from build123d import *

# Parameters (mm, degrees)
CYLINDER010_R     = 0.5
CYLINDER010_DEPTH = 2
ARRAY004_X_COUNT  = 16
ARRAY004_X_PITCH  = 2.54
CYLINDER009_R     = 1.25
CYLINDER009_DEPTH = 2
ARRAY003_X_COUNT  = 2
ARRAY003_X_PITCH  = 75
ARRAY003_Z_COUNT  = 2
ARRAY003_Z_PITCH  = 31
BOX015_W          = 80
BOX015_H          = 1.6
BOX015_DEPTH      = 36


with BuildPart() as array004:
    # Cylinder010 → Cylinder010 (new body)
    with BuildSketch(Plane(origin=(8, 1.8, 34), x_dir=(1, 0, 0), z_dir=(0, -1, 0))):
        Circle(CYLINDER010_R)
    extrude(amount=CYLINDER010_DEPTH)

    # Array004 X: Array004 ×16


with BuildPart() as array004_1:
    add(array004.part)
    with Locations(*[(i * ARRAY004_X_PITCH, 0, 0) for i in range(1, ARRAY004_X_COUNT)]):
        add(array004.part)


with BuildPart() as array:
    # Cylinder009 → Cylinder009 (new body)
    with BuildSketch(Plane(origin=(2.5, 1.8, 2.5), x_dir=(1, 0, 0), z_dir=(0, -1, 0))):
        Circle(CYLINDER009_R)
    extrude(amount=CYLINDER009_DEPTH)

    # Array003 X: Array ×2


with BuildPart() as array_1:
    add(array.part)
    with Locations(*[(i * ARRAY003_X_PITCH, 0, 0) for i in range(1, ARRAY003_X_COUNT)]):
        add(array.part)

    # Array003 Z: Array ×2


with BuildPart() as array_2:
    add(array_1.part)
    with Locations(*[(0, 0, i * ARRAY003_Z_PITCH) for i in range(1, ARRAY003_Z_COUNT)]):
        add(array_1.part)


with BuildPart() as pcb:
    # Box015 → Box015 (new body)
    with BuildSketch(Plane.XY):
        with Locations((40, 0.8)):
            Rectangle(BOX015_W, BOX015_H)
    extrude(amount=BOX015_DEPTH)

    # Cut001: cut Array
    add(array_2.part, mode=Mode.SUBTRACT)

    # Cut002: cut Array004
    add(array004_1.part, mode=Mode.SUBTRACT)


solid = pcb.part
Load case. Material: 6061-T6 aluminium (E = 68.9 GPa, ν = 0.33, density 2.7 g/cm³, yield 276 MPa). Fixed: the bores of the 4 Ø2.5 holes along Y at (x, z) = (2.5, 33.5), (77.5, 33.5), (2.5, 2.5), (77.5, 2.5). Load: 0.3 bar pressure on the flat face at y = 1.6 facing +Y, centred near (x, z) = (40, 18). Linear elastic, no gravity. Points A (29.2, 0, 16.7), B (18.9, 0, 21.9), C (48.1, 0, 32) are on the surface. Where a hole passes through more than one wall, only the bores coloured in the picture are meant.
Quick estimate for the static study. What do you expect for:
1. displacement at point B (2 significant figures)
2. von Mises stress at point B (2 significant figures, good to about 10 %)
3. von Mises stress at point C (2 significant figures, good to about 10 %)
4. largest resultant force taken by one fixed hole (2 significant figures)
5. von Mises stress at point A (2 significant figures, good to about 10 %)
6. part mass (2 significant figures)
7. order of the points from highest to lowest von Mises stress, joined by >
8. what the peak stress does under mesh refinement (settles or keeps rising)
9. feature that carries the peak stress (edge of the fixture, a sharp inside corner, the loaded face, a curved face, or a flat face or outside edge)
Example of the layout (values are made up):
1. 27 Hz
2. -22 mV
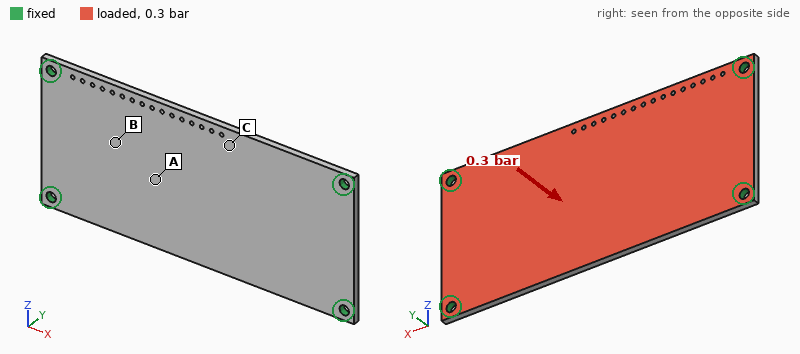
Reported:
1. 0.071 mm
2. 4.8 MPa
3. 17 MPa
4. 21 N
5. 13 MPa
6. 12 g
7. C > A > B
8. keeps rising
9. edge of the fixture
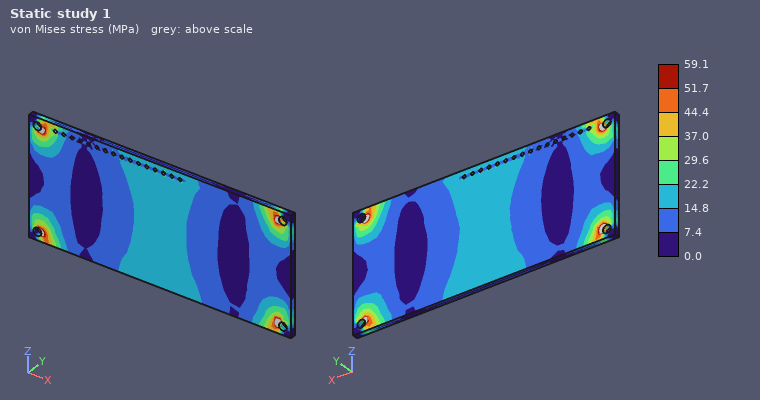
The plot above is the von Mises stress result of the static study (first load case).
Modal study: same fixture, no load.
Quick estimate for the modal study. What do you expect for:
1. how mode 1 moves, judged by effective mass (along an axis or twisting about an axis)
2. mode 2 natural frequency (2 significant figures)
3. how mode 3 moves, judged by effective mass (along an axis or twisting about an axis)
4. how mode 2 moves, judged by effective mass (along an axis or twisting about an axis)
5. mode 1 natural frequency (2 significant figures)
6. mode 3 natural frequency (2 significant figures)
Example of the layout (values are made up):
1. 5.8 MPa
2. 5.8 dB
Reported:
1. along Y
2. 2500 Hz
3. twisting about Z
4. twisting about X
5. 1300 Hz
6. 3700 Hz
